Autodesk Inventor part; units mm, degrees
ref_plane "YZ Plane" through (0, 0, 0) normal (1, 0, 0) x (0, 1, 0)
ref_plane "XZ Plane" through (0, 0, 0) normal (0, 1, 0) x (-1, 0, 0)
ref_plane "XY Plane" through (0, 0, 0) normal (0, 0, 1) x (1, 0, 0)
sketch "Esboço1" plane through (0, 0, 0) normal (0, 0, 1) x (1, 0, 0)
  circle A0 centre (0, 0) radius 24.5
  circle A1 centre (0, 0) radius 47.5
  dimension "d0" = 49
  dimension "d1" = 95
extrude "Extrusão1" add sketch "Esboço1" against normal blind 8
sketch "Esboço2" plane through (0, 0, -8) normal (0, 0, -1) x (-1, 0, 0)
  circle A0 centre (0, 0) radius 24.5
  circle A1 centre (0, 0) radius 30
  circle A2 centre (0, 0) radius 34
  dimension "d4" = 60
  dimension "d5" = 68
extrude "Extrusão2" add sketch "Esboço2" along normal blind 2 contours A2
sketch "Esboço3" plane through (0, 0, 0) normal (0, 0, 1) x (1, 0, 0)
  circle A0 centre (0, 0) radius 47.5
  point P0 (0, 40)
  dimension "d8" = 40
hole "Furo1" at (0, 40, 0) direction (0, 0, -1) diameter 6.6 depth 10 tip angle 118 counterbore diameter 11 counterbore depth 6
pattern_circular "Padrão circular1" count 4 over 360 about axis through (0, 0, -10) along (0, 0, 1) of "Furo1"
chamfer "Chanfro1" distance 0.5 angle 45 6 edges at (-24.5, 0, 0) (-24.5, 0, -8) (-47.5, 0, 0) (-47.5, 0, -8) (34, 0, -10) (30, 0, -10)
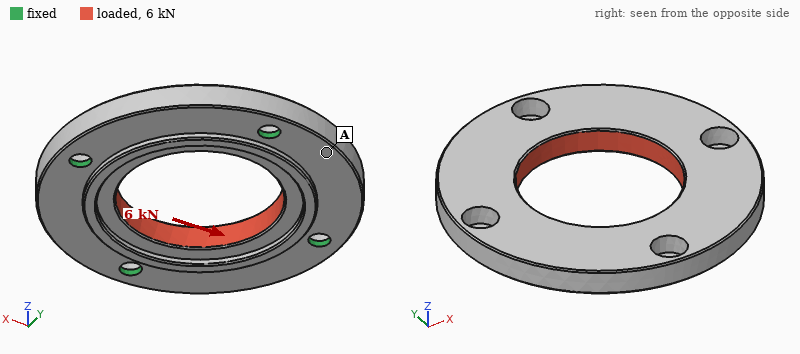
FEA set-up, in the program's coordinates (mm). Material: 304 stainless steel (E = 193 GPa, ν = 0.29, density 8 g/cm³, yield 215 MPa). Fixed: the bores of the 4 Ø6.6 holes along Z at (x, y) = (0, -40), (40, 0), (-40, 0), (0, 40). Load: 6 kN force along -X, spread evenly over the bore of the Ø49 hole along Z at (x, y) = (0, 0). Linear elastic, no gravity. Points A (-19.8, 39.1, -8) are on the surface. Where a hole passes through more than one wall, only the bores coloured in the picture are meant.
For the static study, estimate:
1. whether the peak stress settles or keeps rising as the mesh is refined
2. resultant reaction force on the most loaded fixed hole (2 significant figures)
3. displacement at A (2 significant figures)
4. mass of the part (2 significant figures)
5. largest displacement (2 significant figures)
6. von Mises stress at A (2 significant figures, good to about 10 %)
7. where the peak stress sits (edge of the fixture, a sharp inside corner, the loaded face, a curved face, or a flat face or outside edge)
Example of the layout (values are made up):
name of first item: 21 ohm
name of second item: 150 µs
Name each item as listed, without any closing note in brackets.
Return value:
whether the peak stress settles or keeps rising as the mesh is refined: keeps rising
resultant reaction force on the most loaded fixed hole: 1.5 kN
displacement at A: 2.6 µm
mass of the part: 320 g
largest displacement: 3.7 µm
von Mises stress at A: 8.8 MPa
where the peak stress sits: edge of the fixture
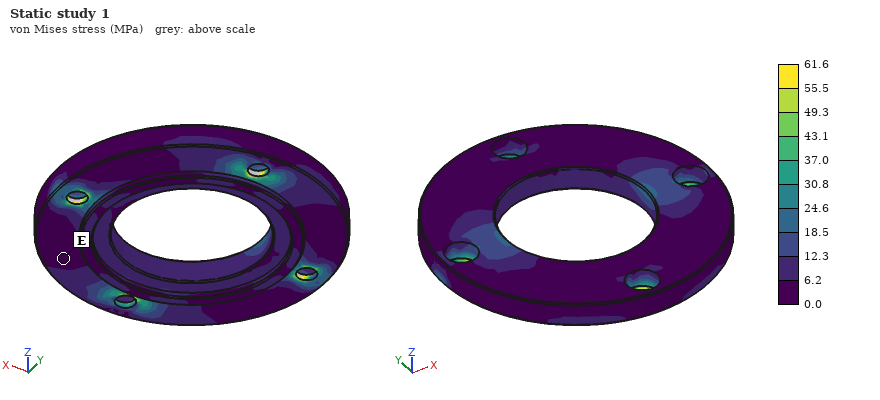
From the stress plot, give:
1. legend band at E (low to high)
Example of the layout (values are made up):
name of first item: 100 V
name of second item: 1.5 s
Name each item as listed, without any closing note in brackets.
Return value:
legend band at E: 0.0 to 6.2 MPa
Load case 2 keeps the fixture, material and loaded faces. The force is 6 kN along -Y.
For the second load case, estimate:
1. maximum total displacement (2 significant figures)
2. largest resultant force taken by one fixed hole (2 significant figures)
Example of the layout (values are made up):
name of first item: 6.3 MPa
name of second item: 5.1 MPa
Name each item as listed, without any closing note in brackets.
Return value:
maximum total displacement: 3.7 µm
largest resultant force taken by one fixed hole: 1.5 kN
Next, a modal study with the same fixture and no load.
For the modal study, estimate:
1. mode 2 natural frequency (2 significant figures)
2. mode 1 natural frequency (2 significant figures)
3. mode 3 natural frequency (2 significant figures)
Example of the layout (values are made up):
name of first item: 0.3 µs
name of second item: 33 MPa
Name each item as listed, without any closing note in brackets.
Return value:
mode 2 natural frequency: 7000 Hz
mode 1 natural frequency: 5500 Hz
mode 3 natural frequency: 7000 Hz
